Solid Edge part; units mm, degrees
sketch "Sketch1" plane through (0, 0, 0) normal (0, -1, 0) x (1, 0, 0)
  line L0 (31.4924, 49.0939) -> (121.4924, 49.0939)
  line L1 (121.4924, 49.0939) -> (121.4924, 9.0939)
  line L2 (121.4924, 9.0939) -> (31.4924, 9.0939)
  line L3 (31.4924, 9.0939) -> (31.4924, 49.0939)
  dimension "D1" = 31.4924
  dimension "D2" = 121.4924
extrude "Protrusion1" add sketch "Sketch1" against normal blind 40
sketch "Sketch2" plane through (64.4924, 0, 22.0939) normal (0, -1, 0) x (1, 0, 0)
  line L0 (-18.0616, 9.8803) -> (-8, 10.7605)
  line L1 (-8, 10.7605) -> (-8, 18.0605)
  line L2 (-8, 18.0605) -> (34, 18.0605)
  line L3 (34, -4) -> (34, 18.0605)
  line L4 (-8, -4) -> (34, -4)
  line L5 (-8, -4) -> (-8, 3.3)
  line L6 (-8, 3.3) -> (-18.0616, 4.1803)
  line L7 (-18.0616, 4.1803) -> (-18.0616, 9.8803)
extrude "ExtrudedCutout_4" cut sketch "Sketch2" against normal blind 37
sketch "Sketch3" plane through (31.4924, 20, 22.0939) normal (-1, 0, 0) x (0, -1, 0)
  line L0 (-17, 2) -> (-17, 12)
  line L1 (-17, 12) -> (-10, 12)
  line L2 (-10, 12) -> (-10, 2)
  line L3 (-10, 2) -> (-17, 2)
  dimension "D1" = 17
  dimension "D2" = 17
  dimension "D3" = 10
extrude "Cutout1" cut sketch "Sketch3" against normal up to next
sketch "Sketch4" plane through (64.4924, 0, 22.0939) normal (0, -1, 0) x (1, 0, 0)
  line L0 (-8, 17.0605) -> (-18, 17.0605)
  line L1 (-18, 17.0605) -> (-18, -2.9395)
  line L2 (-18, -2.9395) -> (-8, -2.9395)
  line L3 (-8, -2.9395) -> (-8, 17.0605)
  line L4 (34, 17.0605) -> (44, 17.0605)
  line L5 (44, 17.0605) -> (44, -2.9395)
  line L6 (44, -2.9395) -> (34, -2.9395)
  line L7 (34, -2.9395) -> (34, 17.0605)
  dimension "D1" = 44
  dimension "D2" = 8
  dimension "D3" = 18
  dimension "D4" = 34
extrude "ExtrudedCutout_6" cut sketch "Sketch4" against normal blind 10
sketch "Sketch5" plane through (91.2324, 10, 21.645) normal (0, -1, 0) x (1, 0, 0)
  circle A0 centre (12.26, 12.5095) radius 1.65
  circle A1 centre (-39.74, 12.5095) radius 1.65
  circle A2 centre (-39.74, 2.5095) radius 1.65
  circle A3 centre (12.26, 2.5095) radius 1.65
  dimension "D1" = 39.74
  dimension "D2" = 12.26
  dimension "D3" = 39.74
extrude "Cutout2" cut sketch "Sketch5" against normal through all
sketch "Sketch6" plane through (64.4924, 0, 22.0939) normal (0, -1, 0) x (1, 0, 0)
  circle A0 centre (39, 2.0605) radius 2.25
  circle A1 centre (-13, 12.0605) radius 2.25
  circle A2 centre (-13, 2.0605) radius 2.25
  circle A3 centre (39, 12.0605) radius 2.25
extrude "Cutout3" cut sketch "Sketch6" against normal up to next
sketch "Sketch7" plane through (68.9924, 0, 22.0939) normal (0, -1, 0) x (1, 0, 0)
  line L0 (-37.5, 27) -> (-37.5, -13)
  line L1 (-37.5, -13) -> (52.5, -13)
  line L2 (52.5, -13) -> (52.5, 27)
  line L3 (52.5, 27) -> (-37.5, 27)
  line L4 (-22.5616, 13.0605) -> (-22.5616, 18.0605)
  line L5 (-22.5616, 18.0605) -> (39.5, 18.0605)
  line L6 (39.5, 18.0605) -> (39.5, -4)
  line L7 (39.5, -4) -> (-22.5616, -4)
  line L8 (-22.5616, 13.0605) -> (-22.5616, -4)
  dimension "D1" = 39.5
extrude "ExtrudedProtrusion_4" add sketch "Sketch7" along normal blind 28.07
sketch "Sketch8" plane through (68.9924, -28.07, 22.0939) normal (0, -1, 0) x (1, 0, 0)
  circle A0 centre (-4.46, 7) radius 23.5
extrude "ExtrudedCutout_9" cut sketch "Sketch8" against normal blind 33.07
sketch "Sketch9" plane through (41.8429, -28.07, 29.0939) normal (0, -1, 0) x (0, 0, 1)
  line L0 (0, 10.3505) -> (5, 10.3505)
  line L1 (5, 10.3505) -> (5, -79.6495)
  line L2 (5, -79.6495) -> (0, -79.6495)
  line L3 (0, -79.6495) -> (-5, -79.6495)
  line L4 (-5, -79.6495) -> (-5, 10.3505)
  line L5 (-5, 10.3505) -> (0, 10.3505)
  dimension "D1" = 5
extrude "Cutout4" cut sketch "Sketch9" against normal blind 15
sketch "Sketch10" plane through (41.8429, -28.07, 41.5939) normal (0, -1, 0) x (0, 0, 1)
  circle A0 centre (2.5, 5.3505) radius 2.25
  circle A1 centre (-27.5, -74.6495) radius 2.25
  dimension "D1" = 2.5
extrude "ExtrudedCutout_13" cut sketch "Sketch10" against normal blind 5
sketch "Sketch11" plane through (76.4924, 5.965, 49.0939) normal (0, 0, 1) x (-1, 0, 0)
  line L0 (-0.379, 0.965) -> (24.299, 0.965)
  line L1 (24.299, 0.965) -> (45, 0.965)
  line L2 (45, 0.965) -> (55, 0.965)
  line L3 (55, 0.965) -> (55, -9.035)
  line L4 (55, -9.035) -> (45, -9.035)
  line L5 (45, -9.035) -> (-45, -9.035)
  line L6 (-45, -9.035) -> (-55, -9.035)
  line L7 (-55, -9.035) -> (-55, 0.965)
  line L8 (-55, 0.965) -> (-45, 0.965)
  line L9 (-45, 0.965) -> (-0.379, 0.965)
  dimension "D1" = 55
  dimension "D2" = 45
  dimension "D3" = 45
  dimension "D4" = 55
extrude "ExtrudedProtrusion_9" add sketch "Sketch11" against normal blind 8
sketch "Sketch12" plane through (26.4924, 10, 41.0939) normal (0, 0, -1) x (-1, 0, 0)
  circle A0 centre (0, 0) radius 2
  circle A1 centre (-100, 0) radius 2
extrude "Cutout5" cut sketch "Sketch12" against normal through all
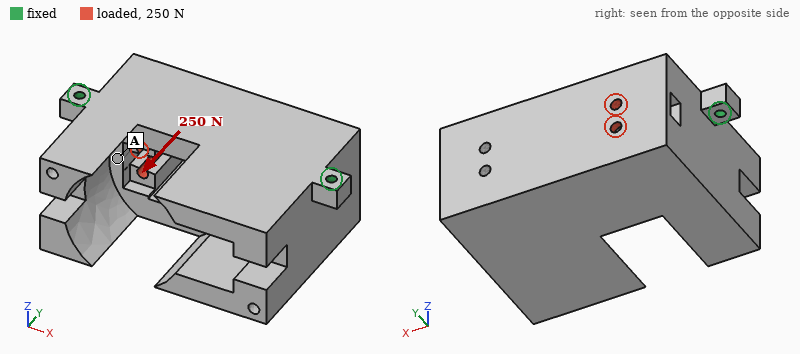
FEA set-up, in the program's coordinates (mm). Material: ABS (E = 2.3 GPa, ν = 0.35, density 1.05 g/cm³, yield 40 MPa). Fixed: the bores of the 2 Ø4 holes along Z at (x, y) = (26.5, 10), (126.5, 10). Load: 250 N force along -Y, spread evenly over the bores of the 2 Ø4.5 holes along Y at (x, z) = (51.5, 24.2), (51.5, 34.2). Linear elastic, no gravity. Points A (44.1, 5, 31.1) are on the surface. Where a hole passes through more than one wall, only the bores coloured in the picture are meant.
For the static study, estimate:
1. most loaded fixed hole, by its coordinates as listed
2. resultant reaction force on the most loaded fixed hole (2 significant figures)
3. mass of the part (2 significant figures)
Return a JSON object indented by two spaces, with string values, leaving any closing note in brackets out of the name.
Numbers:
{
  "most loaded fixed hole, by its coordinates as listed": "(26.5, 10)",
  "resultant reaction force on the most loaded fixed hole": "200 N",
  "mass of the part": "140 g"
}
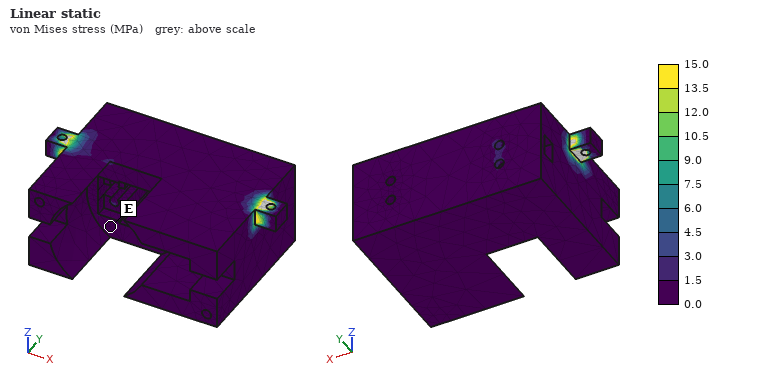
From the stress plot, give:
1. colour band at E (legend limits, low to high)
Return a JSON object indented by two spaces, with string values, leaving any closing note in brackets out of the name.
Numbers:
{
  "colour band at E": "0.0 to 1.5 MPa"
}
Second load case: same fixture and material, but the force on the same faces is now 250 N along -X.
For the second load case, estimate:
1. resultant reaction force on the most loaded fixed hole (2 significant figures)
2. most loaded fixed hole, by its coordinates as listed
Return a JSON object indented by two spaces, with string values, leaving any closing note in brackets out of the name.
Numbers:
{
  "resultant reaction force on the most loaded fixed hole": "150 N",
  "most loaded fixed hole, by its coordinates as listed": "(26.5, 10)"
}
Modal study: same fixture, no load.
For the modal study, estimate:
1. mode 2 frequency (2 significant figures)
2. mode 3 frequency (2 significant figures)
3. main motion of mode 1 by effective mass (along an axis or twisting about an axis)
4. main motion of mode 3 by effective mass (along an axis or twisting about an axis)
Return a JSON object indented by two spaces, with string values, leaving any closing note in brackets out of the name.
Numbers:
{
  "mode 2 frequency": "900 Hz",
  "mode 3 frequency": "1300 Hz",
  "main motion of mode 1 by effective mass": "along Y",
  "main motion of mode 3 by effective mass": "along Z"
}
